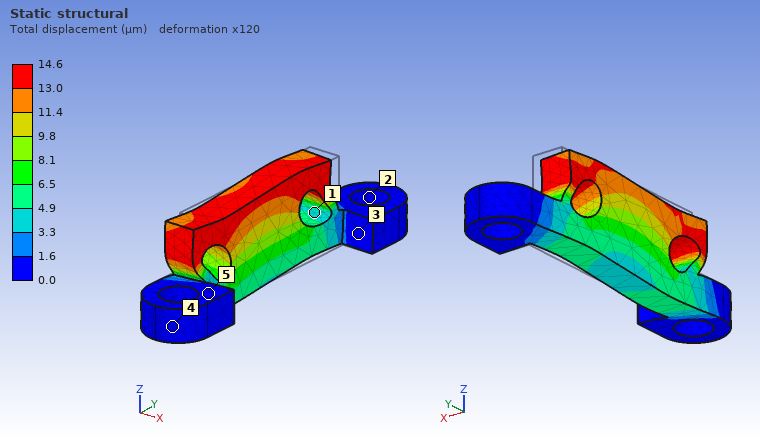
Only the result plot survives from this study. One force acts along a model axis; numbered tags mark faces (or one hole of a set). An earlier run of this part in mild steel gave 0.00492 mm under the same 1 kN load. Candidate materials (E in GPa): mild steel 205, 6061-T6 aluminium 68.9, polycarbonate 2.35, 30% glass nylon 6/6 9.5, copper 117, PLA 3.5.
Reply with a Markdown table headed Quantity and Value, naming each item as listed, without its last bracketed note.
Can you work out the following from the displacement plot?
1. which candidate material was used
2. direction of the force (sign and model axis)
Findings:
| Quantity | Value |
|---|---|
| which candidate material was used | 6061-T6 aluminium |
| direction of the force | -Y |
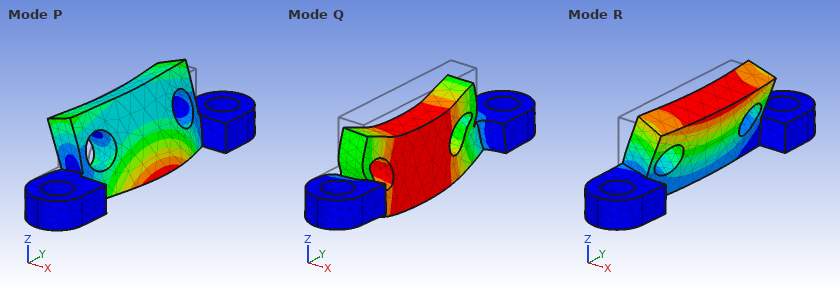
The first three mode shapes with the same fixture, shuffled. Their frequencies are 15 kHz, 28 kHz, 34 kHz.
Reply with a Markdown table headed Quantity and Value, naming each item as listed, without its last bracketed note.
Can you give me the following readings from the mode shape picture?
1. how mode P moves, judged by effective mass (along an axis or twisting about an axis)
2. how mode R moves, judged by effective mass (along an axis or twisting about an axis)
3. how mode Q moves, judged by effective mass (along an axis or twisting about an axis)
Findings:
| Quantity | Value |
|---|---|
| how mode P moves, judged by effective mass | along X |
| how mode R moves, judged by effective mass | along X |
| how mode Q moves, judged by effective mass | along Z |
